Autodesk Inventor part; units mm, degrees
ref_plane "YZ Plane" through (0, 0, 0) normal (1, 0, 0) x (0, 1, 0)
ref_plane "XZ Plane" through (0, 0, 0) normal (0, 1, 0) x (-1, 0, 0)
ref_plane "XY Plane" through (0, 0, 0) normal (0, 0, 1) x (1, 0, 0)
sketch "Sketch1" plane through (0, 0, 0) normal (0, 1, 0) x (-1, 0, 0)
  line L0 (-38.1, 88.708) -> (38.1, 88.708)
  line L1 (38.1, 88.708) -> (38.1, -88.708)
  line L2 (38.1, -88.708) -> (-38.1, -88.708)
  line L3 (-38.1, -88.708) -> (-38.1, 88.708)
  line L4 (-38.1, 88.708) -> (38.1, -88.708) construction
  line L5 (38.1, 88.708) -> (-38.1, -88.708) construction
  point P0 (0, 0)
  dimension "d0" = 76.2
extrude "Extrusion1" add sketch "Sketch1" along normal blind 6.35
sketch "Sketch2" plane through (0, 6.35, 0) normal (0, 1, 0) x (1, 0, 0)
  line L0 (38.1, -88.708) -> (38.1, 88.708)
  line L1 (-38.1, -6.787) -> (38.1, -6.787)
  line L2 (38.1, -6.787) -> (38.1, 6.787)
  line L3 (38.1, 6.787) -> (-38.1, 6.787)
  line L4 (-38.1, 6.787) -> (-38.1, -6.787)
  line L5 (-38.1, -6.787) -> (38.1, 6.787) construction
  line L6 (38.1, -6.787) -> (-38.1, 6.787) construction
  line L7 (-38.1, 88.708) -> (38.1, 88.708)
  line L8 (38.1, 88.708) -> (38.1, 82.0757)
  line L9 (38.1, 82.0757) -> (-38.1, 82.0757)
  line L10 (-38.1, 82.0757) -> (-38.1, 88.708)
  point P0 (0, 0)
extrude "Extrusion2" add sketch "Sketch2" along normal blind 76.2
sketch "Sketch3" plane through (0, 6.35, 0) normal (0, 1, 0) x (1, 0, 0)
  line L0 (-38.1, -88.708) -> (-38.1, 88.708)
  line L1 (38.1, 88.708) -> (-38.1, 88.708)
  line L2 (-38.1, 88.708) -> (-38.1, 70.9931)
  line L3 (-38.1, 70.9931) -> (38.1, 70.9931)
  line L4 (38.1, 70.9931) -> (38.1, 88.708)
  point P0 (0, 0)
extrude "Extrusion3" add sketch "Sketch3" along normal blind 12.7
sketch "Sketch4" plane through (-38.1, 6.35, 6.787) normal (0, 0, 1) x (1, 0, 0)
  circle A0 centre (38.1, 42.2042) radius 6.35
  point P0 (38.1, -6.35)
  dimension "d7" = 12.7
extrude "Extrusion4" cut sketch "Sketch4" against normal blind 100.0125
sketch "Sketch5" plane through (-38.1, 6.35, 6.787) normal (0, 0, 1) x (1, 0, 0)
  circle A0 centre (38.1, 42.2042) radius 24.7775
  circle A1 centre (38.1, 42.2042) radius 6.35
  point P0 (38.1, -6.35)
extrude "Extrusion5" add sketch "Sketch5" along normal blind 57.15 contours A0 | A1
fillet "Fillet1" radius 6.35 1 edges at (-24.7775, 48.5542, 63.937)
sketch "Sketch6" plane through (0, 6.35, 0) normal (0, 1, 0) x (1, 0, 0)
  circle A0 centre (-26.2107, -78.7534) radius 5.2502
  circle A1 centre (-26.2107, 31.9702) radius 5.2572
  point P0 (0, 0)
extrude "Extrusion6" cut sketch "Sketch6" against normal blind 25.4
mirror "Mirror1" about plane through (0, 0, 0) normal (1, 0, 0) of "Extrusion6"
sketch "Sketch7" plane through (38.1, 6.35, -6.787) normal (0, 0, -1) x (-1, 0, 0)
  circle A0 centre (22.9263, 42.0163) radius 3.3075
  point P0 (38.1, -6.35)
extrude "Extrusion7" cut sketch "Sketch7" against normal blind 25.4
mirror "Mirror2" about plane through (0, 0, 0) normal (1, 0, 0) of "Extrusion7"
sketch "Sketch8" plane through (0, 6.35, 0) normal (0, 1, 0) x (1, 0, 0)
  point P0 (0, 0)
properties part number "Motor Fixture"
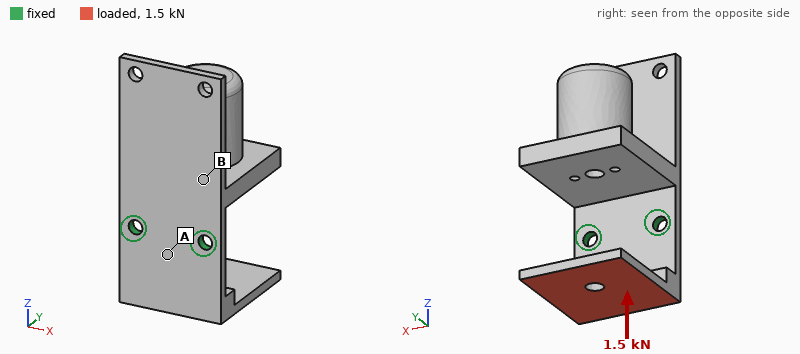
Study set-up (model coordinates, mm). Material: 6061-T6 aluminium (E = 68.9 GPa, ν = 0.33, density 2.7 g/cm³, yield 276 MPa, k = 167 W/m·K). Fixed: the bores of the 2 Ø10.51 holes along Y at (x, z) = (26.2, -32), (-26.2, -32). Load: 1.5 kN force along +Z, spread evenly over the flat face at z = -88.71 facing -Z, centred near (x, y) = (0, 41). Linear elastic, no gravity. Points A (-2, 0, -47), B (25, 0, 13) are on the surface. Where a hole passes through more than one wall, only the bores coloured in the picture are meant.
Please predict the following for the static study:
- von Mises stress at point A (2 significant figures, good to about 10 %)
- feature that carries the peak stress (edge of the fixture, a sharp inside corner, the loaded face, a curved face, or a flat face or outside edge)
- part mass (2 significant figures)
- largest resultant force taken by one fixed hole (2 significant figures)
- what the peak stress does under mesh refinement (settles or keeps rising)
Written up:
83 MPa
edge of the fixture
850 g
770 N
keeps rising
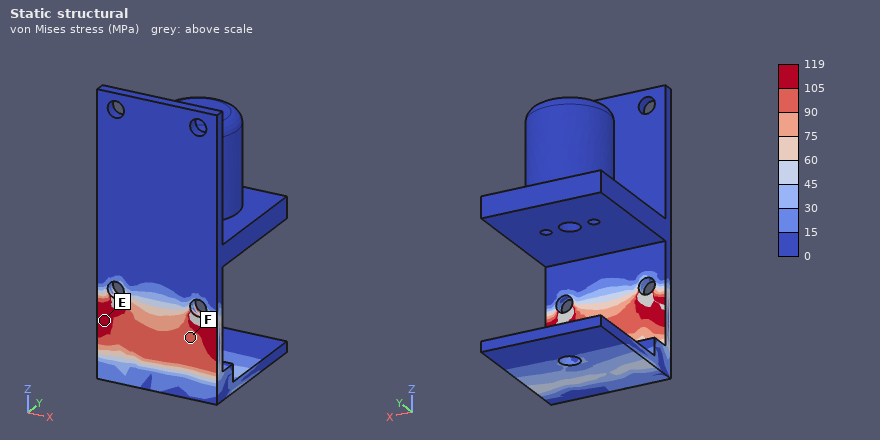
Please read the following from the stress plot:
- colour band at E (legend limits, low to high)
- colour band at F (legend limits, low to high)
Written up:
105 to 119 MPa
90 to 105 MPa
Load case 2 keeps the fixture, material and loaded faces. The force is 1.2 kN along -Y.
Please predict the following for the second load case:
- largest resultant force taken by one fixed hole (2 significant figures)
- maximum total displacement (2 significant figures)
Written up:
600 N
1.3 mm
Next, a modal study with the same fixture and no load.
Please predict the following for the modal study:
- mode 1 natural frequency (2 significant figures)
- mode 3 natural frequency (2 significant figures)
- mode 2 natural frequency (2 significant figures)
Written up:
210 Hz
810 Hz
440 Hz
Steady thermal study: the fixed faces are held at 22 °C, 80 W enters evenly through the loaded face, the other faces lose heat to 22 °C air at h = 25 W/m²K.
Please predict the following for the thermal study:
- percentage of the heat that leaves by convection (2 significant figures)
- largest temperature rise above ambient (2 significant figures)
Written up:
21 %
62 K
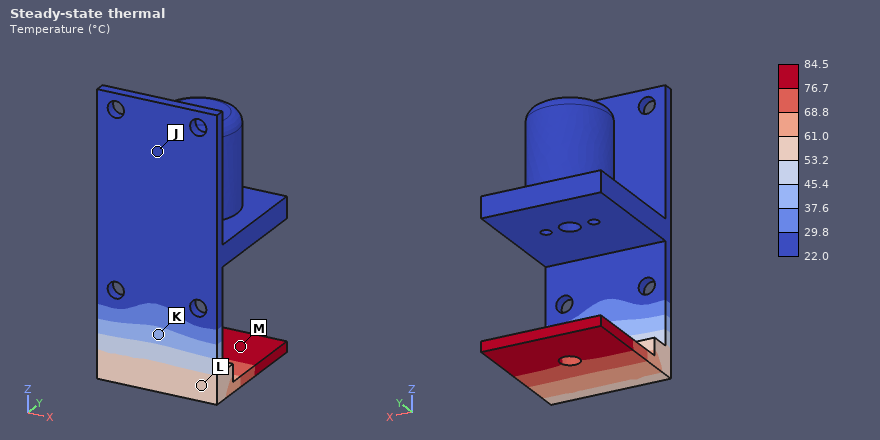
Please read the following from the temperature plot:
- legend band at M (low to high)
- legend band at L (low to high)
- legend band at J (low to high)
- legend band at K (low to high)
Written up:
76.7 to 84.5 °C
53.2 to 61.0 °C
22.0 to 29.8 °C
37.6 to 45.4 °C
